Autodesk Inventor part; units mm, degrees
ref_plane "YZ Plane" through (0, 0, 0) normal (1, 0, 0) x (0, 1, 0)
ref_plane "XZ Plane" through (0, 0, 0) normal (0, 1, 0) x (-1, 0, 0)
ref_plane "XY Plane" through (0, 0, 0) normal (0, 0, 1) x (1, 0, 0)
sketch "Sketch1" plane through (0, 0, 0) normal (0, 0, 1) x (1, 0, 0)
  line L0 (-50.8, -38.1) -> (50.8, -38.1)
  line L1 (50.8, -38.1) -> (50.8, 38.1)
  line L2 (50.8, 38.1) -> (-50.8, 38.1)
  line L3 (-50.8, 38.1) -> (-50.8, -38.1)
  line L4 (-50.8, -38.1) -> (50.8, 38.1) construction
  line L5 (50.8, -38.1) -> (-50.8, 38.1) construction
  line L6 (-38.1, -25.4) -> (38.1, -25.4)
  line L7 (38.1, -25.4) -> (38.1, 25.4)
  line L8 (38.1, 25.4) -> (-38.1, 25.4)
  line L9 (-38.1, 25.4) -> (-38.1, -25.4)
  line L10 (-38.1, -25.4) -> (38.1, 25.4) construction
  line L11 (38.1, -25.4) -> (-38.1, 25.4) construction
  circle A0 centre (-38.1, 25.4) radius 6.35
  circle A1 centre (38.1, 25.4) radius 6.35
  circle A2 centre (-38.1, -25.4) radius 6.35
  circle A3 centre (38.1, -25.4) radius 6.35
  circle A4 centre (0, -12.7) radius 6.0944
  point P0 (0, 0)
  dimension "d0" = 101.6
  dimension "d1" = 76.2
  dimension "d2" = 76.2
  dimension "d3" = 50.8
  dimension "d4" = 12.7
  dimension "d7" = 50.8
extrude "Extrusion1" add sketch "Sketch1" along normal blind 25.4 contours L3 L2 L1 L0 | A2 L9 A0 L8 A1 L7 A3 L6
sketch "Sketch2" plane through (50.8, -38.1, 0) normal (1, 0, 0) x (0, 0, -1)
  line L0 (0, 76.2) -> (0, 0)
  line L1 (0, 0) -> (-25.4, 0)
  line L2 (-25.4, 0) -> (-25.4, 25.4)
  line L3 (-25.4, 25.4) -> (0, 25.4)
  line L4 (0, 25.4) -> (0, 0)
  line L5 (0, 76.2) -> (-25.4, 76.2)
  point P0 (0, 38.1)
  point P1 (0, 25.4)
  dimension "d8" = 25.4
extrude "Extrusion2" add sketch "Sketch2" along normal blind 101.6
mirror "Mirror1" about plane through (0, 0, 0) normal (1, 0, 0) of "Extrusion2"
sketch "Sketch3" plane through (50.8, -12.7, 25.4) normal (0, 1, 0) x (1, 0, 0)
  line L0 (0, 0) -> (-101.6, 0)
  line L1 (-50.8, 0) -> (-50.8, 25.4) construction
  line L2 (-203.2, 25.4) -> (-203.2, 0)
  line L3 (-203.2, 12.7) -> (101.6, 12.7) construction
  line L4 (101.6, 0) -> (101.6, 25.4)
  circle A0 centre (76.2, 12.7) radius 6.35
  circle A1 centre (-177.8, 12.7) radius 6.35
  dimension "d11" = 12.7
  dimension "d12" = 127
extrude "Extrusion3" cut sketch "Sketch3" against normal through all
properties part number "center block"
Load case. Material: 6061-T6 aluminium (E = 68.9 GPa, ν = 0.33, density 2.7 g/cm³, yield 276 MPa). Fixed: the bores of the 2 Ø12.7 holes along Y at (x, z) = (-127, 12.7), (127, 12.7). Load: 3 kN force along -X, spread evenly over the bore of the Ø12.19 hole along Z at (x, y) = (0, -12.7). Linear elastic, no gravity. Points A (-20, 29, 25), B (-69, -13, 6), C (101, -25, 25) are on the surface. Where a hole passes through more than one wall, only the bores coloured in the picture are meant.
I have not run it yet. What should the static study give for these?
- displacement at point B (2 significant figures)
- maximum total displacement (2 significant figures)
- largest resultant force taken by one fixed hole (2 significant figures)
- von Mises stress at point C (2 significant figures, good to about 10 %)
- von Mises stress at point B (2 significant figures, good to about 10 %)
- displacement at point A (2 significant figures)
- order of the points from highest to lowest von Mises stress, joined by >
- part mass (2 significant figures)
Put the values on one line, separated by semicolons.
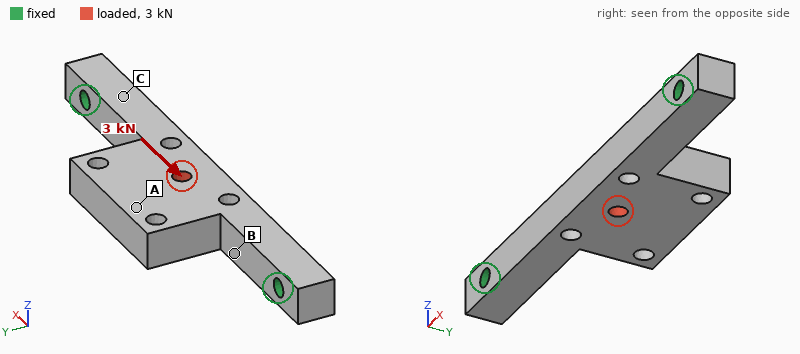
2.8 µm; 7.4 µm; 1.5 kN; 2.5 MPa; 4.1 MPa; 6.5 µm; B > C > A; 820 g
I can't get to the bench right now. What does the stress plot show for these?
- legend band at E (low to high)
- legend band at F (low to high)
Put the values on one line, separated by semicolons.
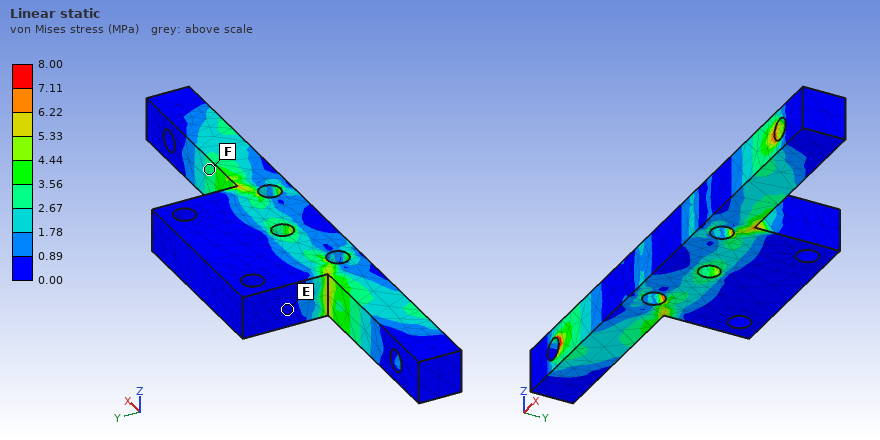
0.00 to 0.89 MPa; 2.67 to 3.56 MPa
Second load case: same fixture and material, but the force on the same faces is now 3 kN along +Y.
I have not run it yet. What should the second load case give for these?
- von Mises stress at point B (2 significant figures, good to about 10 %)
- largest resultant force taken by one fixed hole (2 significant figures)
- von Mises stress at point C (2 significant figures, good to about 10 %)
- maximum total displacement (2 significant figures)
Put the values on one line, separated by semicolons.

6.9 MPa; 1.7 kN; 6.9 MPa; 48 µm
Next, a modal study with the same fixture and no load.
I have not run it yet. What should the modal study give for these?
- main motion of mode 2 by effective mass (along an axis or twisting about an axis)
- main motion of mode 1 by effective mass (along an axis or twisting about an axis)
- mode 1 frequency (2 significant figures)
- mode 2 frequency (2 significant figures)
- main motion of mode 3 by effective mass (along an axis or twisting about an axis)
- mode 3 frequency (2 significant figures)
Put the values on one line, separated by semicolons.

along Y; along Z; 970 Hz; 1800 Hz; along Z; 2300 Hz
